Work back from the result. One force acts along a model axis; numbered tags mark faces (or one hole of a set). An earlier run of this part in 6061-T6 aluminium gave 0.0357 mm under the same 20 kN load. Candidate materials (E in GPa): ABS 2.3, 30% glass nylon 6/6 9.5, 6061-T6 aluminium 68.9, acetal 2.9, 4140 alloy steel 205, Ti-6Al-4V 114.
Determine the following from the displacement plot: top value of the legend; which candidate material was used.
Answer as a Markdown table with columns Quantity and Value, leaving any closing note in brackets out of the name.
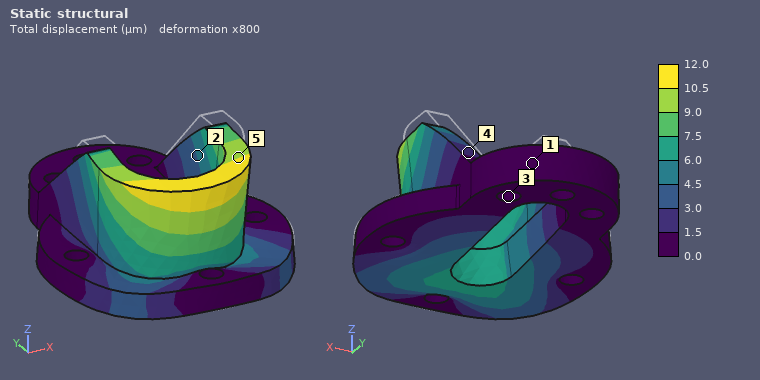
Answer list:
| Quantity | Value |
|---|---|
| top value of the legend | 12.0 µm |
| which candidate material was used | 4140 alloy steel |
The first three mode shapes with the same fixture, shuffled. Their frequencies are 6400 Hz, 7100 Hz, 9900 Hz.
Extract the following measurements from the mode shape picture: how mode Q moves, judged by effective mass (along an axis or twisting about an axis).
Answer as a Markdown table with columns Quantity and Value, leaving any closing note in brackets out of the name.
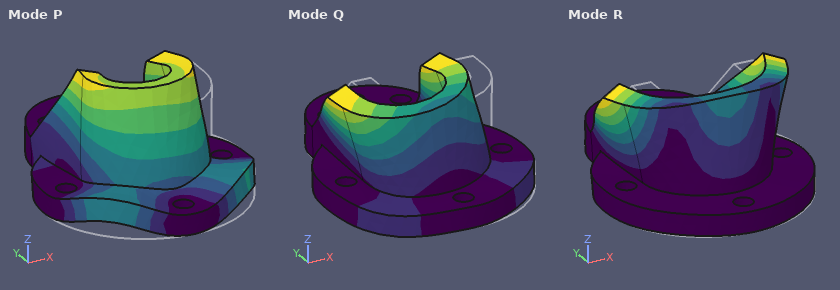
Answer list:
| Quantity | Value |
|---|---|
| how mode Q moves, judged by effective mass | along X |
